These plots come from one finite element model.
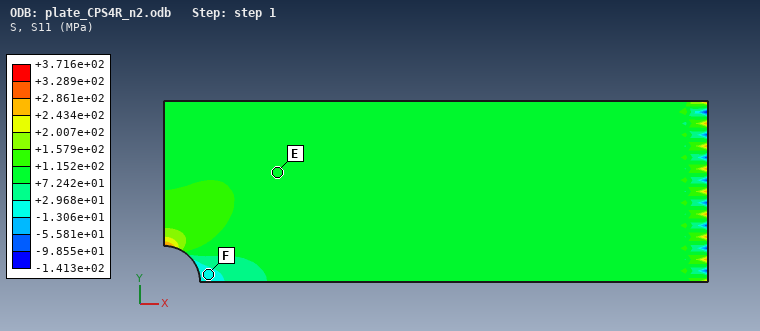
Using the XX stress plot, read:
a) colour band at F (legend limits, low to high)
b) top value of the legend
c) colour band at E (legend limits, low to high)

-1.306e+01 to +2.968e+01 MPa
+3.716e+02 MPa
+7.242e+01 to +1.152e+02 MPa
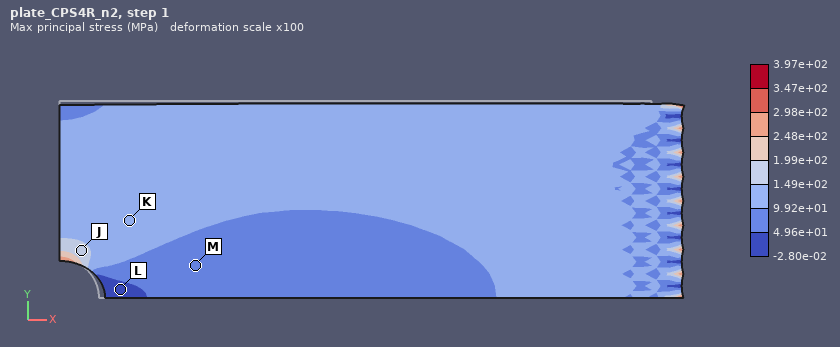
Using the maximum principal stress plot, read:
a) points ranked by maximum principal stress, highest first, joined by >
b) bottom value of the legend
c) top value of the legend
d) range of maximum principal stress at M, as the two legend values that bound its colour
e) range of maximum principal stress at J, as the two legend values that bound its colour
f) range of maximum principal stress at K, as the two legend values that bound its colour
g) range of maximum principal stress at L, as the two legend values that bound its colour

J > K > M > L
-2.80e-02 MPa
3.97e+02 MPa
4.96e+01 to 9.92e+01 MPa
1.49e+02 to 1.99e+02 MPa
9.92e+01 to 1.49e+02 MPa
-2.80e-02 to 4.96e+01 MPa
